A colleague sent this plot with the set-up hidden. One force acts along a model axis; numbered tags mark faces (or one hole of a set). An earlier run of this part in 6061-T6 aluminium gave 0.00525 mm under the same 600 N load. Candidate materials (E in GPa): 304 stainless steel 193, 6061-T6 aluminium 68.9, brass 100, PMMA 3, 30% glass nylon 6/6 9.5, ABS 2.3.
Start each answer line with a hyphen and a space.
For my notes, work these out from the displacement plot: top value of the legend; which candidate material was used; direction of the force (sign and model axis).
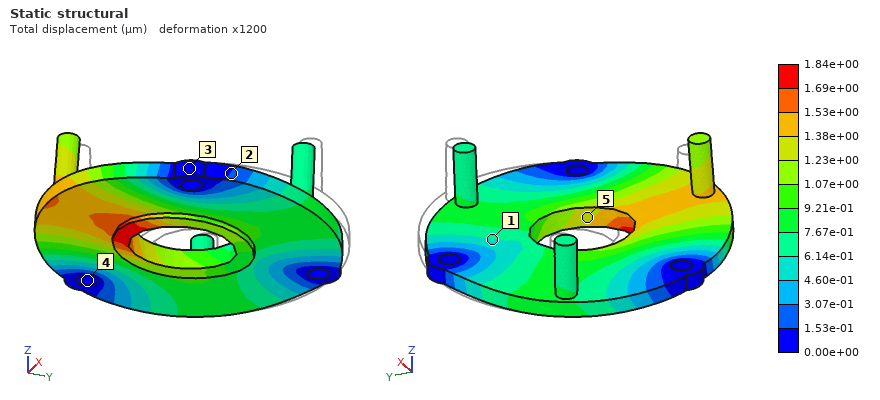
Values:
- 1.84e+00 µm
- 304 stainless steel
- -Y
